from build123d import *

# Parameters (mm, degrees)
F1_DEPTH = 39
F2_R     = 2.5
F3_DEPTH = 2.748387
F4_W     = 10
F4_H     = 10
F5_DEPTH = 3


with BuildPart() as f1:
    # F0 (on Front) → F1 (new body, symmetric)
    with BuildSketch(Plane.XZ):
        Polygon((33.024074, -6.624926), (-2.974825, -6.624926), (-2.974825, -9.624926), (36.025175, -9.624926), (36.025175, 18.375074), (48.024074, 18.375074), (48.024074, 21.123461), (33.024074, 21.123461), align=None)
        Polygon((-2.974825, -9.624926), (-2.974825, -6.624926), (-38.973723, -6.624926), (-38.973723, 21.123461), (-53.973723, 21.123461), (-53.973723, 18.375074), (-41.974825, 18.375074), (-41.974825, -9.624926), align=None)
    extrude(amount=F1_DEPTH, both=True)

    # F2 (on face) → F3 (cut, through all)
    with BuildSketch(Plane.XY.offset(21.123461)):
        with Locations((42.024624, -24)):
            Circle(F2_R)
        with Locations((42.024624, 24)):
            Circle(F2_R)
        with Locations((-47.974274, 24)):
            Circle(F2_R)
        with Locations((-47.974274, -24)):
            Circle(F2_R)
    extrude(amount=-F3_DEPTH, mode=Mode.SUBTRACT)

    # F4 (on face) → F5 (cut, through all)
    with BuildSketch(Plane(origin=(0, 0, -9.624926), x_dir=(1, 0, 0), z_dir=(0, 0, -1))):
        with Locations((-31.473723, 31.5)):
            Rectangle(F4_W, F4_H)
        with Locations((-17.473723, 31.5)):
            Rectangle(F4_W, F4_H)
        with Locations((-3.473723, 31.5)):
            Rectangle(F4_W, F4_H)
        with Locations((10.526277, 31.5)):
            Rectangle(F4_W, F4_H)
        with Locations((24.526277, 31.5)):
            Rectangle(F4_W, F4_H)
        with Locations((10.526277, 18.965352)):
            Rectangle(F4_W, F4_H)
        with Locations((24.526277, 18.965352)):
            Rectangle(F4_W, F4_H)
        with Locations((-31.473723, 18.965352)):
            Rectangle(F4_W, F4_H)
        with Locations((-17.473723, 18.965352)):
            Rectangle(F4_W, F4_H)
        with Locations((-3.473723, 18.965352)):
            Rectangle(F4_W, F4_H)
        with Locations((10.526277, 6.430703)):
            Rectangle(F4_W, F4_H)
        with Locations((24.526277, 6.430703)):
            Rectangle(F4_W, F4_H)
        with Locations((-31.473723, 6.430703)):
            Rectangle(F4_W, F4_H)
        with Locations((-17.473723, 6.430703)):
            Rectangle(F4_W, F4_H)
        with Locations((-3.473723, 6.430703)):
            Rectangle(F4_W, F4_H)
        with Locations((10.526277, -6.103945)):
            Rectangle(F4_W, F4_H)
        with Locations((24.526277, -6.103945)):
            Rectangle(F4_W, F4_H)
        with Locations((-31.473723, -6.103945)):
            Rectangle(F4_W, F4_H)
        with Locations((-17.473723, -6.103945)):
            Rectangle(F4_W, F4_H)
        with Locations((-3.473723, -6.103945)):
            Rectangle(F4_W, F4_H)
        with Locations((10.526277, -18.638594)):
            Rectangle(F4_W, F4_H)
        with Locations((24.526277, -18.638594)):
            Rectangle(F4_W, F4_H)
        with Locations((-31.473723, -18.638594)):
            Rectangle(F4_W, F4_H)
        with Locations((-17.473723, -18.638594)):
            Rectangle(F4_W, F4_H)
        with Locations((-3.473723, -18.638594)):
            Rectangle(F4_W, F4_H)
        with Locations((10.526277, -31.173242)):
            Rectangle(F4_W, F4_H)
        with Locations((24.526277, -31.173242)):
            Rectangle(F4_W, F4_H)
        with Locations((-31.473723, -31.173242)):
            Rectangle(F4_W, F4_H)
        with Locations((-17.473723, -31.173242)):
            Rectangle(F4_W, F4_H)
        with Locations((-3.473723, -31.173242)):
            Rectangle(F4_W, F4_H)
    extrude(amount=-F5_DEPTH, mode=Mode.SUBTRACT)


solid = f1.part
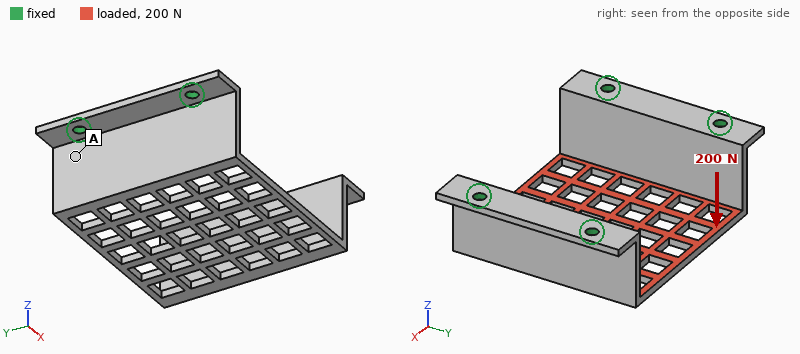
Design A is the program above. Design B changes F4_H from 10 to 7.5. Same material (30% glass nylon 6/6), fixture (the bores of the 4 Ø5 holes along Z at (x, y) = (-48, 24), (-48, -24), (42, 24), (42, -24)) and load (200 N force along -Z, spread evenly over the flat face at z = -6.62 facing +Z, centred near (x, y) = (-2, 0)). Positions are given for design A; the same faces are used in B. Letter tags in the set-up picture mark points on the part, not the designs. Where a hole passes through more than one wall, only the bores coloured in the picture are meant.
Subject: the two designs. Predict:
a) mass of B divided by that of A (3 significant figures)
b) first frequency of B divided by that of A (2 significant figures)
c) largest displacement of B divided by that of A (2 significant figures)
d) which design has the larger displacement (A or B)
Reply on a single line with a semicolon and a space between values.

1.08; 1.0; 0.67; A
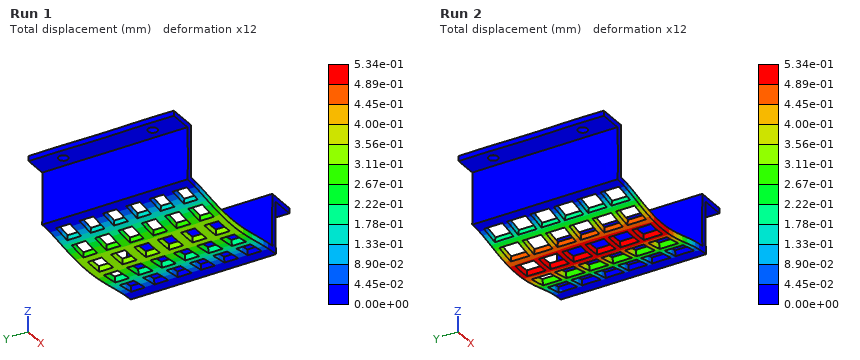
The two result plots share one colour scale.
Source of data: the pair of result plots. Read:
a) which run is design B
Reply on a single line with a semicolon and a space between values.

Run 1
